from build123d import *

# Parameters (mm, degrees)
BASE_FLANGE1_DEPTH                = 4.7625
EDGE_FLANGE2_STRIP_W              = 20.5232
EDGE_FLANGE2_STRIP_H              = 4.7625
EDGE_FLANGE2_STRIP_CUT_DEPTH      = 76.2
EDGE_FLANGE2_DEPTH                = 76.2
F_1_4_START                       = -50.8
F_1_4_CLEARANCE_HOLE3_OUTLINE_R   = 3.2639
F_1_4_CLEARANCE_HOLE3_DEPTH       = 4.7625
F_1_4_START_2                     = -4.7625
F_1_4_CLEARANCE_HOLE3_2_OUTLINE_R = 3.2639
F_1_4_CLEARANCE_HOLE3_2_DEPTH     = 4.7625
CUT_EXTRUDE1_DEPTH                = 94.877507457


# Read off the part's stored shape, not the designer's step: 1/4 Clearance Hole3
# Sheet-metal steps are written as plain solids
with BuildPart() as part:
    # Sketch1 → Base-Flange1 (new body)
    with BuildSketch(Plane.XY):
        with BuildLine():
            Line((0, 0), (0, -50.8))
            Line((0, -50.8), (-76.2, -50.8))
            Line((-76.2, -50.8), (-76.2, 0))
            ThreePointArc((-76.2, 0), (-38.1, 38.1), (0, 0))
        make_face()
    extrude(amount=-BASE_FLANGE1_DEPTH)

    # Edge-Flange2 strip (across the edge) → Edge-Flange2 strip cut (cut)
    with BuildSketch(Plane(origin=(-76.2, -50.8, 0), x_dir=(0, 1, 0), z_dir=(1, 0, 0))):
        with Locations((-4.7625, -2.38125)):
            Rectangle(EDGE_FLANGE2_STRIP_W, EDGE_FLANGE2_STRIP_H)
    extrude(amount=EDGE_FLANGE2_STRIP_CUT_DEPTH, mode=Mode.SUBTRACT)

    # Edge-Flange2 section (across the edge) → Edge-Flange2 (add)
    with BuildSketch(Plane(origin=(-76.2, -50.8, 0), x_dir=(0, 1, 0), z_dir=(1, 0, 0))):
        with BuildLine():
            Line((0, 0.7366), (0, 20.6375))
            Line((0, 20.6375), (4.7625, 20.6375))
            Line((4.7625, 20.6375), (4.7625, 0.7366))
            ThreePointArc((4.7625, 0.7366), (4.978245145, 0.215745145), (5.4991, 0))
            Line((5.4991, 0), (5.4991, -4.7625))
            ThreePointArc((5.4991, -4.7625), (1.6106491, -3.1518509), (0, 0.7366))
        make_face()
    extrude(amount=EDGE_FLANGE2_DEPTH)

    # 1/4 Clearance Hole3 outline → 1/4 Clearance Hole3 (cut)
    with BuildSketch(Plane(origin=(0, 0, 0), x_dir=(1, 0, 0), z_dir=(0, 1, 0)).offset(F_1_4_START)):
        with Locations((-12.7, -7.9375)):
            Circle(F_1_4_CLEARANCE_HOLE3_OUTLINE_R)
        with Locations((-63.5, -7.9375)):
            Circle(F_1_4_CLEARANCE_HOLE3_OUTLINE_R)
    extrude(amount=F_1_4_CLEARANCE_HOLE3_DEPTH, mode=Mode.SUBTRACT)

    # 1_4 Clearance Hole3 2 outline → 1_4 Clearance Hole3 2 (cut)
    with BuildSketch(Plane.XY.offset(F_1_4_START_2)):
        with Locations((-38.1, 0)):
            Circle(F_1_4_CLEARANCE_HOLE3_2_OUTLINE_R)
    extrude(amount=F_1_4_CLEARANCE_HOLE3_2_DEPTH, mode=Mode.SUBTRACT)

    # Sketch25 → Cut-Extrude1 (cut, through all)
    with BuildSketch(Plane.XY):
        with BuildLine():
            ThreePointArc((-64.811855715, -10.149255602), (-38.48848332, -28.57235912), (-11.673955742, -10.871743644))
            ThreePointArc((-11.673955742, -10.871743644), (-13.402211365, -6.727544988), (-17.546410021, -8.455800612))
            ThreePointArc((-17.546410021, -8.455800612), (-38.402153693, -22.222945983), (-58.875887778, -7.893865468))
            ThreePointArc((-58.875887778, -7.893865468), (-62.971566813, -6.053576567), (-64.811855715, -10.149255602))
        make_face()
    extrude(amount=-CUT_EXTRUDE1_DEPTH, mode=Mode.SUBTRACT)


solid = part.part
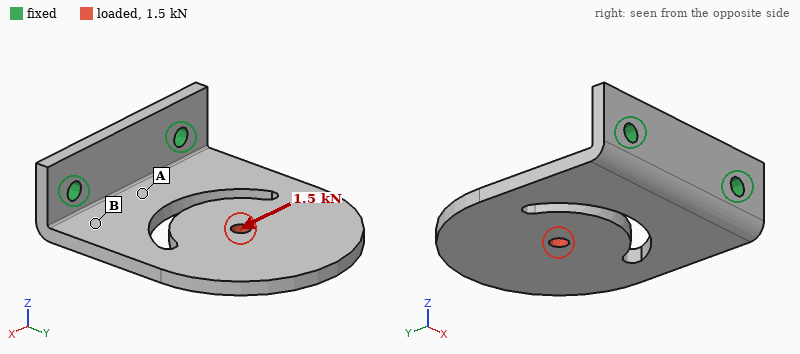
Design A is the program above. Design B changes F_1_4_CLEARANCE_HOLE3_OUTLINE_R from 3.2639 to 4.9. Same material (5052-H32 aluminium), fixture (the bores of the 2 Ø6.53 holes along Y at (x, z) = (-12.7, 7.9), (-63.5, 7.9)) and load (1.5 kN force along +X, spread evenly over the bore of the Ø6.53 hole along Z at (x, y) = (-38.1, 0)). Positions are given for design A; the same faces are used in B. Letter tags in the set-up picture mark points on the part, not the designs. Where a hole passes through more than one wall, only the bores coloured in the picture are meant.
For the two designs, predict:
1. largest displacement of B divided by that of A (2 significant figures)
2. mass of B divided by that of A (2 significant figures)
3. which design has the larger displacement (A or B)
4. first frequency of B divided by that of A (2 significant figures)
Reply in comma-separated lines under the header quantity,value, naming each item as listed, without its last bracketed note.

quantity,value
largest displacement of B divided by that of A,0.77
mass of B divided by that of A,0.99
which design has the larger displacement,A
first frequency of B divided by that of A,1.0
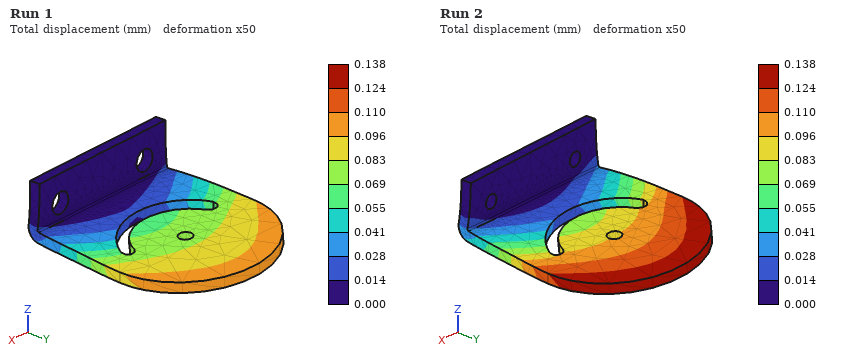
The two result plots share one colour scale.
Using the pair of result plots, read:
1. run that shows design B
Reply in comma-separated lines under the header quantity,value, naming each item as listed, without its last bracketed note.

quantity,value
run that shows design B,Run 1
